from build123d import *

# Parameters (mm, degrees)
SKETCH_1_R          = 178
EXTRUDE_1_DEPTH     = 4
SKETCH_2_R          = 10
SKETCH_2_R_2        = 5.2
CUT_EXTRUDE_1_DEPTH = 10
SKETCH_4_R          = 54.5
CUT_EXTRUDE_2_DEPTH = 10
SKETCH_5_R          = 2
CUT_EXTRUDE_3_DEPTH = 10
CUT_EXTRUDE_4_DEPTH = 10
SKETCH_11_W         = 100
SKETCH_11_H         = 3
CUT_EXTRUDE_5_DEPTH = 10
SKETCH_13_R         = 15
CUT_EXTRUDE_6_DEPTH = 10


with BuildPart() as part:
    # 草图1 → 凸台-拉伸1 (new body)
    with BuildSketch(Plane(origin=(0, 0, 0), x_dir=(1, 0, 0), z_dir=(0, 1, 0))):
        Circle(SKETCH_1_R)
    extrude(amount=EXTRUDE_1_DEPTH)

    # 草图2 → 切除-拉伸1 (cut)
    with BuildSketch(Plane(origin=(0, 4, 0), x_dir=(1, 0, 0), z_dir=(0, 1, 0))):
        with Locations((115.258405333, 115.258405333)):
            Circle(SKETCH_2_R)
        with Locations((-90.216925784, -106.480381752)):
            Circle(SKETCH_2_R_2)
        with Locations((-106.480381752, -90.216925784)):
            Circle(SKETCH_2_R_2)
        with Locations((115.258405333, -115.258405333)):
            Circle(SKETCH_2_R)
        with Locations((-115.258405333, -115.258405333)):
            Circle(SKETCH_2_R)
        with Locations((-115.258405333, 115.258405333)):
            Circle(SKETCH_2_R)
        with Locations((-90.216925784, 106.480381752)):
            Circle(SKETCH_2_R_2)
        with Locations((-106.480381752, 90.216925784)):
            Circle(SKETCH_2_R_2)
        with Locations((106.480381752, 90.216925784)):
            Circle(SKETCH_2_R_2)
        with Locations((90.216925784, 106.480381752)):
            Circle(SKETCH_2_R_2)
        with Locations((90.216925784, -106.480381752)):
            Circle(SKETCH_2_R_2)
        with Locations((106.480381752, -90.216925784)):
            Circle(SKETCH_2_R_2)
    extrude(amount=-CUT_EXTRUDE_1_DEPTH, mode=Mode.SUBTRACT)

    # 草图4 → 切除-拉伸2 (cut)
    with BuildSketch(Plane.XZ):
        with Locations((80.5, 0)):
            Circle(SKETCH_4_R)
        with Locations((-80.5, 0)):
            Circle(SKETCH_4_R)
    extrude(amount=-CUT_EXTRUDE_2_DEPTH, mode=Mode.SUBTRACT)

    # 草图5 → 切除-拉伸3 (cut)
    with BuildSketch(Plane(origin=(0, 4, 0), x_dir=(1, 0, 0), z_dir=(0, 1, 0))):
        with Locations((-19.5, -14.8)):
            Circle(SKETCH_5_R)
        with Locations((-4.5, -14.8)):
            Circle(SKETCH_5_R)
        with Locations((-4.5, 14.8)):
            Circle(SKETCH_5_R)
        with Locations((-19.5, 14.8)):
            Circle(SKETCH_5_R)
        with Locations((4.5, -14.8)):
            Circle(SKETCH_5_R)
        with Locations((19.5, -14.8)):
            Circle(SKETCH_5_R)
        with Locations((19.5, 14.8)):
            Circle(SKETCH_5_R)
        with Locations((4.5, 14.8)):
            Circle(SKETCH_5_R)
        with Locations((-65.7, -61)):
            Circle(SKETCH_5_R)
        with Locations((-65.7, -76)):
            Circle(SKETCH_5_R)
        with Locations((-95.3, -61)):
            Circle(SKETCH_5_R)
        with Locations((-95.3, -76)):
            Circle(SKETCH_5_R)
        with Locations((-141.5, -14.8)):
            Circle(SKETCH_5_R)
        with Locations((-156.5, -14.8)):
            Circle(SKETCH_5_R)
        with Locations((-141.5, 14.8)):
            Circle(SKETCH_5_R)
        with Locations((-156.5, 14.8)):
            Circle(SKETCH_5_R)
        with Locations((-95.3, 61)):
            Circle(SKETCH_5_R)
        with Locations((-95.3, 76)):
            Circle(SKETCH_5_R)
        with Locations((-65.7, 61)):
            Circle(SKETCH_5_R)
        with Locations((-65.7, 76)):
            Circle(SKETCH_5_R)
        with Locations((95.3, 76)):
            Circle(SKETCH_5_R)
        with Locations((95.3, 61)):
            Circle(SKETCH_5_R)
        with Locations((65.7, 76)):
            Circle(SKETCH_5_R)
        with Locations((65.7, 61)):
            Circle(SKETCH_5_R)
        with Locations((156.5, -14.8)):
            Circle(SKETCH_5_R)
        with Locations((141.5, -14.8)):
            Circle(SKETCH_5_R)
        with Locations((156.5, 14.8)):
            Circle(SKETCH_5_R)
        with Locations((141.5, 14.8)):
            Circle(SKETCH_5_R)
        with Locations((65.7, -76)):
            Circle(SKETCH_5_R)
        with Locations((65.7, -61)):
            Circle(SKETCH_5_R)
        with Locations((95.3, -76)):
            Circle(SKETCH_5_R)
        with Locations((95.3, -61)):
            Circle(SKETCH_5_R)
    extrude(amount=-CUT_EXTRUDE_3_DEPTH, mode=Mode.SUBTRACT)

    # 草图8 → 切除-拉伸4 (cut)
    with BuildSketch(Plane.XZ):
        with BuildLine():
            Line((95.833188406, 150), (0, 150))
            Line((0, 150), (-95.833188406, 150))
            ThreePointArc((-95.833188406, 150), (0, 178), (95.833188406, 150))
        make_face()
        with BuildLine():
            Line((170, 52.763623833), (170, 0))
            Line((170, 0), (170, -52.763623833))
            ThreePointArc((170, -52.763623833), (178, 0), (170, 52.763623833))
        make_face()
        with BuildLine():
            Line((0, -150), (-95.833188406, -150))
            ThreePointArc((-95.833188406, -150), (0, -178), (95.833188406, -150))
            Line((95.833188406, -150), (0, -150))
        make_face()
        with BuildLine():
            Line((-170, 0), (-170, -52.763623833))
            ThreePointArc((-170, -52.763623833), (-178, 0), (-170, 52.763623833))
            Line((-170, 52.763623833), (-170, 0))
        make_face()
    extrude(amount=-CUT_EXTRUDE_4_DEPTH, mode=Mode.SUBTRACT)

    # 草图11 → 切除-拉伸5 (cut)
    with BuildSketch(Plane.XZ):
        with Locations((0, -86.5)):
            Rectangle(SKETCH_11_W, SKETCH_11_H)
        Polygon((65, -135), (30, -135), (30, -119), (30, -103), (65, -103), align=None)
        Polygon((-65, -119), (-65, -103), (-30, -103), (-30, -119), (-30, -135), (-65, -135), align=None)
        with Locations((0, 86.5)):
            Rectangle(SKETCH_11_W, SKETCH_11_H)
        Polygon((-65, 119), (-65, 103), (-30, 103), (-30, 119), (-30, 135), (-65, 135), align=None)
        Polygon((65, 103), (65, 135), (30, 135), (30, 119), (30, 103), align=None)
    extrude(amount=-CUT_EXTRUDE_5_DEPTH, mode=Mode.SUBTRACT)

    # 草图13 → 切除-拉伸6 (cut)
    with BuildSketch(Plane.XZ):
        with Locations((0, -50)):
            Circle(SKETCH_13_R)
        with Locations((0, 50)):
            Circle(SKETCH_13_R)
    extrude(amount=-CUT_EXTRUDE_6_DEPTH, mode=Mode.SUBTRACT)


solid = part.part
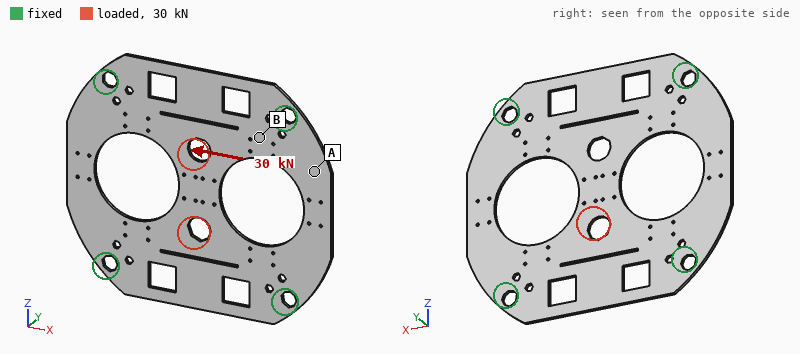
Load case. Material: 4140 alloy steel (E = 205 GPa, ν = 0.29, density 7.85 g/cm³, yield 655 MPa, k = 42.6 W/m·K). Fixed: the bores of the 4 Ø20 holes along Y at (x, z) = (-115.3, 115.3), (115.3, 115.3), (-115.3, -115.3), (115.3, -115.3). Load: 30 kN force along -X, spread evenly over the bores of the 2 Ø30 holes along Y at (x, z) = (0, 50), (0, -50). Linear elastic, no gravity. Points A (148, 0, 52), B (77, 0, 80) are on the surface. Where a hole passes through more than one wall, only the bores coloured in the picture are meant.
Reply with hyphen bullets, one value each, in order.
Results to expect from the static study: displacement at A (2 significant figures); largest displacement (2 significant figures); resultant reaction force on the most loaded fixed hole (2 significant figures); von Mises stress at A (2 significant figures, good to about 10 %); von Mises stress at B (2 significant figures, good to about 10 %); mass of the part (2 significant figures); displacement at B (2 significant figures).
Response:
- 13 µm
- 40 µm
- 7.8 kN
- 12 MPa
- 40 MPa
- 2.0 kg
- 14 µm
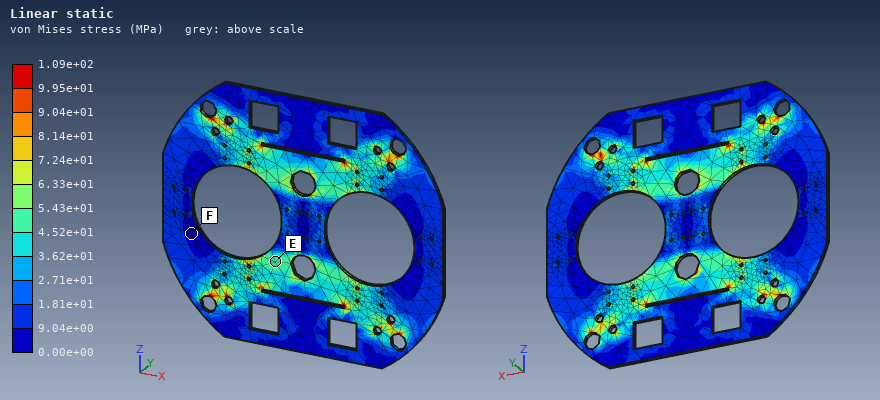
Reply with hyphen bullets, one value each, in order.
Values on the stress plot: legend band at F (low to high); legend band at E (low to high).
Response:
- 0.00e+00 to 9.04e+00 MPa
- 4.52e+01 to 5.43e+01 MPa
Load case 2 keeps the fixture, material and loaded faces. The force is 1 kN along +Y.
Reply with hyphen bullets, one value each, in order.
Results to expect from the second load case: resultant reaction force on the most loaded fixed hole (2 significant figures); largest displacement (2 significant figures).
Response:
- 250 N
- 0.77 mm
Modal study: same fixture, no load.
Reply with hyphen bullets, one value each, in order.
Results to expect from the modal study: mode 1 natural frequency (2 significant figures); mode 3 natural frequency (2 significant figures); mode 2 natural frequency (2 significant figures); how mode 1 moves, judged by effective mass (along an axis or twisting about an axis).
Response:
- 300 Hz
- 420 Hz
- 410 Hz
- along Y
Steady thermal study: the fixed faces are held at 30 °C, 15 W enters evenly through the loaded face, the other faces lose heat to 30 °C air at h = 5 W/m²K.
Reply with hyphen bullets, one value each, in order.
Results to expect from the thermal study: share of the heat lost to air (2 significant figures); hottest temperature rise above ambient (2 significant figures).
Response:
- 48 %
- 39 K
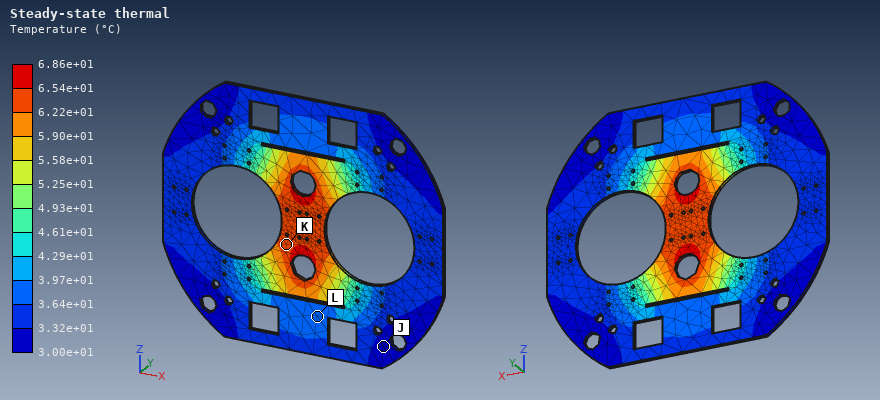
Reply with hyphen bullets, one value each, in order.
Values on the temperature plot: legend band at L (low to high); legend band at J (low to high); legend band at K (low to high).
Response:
- 3.64e+01 to 3.97e+01 °C
- 3.00e+01 to 3.32e+01 °C
- 6.22e+01 to 6.54e+01 °C
